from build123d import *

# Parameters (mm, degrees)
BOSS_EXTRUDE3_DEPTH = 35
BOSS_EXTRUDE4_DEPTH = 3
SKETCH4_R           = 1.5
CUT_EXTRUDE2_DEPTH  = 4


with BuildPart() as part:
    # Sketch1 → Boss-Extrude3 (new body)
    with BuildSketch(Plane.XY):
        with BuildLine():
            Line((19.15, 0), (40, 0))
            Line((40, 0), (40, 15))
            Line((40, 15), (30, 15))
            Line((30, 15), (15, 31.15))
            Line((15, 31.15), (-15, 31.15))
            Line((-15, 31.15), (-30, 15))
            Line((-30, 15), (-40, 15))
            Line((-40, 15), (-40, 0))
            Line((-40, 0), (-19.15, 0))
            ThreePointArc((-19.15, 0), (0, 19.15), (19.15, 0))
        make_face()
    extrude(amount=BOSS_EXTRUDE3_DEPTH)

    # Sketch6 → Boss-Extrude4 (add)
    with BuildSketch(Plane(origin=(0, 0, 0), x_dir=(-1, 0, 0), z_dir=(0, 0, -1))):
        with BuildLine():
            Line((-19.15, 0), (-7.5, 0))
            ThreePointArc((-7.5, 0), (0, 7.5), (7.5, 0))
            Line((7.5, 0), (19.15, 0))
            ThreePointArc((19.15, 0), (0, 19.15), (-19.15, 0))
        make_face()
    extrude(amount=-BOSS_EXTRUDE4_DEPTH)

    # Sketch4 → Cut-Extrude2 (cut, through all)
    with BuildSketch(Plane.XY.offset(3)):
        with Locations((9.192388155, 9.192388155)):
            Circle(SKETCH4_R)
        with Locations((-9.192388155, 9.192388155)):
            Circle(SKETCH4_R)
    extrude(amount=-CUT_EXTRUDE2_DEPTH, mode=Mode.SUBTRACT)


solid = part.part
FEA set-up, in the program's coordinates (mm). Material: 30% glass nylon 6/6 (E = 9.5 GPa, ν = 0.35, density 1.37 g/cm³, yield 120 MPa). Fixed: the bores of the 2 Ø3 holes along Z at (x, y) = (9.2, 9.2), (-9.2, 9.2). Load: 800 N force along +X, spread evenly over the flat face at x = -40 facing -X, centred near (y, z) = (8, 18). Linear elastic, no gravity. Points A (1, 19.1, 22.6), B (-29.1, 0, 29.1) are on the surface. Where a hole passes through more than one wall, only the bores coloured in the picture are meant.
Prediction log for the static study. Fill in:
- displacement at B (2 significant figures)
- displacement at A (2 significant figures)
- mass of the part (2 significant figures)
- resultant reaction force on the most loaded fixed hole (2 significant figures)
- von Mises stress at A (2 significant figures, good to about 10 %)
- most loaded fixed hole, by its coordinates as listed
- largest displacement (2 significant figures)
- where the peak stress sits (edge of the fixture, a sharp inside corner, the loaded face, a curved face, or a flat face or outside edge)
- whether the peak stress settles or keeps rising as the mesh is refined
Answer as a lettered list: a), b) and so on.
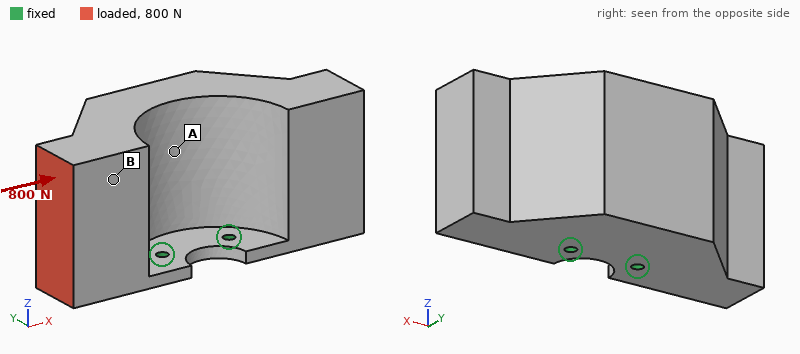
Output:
a) 0.45 mm
b) 0.20 mm
c) 67 g
d) 800 N
e) 11 MPa
f) (-9.2, 9.2)
g) 0.58 mm
h) edge of the fixture
i) keeps rising
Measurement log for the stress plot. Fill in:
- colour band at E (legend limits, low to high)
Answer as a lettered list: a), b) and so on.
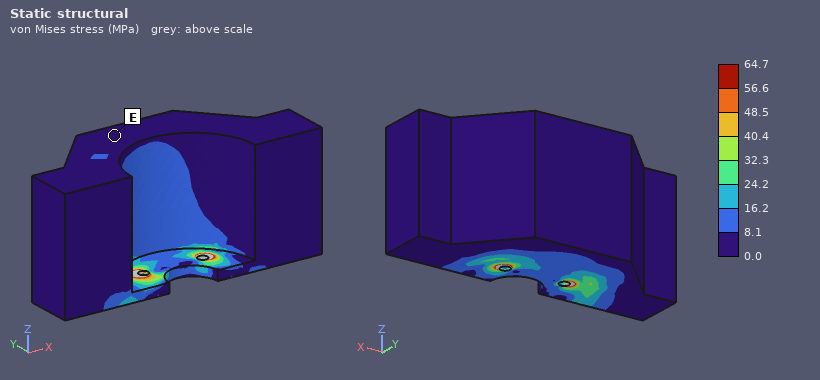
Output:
a) 0.0 to 8.1 MPa
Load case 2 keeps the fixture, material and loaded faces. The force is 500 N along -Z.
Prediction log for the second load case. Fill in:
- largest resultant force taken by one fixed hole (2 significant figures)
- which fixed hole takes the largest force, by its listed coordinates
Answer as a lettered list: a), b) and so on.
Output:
a) 1.1 kN
b) (-9.2, 9.2)
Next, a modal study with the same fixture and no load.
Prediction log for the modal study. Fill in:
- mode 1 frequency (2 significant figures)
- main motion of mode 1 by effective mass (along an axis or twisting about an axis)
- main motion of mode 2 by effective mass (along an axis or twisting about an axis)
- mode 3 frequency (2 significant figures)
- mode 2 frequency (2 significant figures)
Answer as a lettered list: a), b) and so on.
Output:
a) 430 Hz
b) along Y
c) along X
d) 1600 Hz
e) 830 Hz
